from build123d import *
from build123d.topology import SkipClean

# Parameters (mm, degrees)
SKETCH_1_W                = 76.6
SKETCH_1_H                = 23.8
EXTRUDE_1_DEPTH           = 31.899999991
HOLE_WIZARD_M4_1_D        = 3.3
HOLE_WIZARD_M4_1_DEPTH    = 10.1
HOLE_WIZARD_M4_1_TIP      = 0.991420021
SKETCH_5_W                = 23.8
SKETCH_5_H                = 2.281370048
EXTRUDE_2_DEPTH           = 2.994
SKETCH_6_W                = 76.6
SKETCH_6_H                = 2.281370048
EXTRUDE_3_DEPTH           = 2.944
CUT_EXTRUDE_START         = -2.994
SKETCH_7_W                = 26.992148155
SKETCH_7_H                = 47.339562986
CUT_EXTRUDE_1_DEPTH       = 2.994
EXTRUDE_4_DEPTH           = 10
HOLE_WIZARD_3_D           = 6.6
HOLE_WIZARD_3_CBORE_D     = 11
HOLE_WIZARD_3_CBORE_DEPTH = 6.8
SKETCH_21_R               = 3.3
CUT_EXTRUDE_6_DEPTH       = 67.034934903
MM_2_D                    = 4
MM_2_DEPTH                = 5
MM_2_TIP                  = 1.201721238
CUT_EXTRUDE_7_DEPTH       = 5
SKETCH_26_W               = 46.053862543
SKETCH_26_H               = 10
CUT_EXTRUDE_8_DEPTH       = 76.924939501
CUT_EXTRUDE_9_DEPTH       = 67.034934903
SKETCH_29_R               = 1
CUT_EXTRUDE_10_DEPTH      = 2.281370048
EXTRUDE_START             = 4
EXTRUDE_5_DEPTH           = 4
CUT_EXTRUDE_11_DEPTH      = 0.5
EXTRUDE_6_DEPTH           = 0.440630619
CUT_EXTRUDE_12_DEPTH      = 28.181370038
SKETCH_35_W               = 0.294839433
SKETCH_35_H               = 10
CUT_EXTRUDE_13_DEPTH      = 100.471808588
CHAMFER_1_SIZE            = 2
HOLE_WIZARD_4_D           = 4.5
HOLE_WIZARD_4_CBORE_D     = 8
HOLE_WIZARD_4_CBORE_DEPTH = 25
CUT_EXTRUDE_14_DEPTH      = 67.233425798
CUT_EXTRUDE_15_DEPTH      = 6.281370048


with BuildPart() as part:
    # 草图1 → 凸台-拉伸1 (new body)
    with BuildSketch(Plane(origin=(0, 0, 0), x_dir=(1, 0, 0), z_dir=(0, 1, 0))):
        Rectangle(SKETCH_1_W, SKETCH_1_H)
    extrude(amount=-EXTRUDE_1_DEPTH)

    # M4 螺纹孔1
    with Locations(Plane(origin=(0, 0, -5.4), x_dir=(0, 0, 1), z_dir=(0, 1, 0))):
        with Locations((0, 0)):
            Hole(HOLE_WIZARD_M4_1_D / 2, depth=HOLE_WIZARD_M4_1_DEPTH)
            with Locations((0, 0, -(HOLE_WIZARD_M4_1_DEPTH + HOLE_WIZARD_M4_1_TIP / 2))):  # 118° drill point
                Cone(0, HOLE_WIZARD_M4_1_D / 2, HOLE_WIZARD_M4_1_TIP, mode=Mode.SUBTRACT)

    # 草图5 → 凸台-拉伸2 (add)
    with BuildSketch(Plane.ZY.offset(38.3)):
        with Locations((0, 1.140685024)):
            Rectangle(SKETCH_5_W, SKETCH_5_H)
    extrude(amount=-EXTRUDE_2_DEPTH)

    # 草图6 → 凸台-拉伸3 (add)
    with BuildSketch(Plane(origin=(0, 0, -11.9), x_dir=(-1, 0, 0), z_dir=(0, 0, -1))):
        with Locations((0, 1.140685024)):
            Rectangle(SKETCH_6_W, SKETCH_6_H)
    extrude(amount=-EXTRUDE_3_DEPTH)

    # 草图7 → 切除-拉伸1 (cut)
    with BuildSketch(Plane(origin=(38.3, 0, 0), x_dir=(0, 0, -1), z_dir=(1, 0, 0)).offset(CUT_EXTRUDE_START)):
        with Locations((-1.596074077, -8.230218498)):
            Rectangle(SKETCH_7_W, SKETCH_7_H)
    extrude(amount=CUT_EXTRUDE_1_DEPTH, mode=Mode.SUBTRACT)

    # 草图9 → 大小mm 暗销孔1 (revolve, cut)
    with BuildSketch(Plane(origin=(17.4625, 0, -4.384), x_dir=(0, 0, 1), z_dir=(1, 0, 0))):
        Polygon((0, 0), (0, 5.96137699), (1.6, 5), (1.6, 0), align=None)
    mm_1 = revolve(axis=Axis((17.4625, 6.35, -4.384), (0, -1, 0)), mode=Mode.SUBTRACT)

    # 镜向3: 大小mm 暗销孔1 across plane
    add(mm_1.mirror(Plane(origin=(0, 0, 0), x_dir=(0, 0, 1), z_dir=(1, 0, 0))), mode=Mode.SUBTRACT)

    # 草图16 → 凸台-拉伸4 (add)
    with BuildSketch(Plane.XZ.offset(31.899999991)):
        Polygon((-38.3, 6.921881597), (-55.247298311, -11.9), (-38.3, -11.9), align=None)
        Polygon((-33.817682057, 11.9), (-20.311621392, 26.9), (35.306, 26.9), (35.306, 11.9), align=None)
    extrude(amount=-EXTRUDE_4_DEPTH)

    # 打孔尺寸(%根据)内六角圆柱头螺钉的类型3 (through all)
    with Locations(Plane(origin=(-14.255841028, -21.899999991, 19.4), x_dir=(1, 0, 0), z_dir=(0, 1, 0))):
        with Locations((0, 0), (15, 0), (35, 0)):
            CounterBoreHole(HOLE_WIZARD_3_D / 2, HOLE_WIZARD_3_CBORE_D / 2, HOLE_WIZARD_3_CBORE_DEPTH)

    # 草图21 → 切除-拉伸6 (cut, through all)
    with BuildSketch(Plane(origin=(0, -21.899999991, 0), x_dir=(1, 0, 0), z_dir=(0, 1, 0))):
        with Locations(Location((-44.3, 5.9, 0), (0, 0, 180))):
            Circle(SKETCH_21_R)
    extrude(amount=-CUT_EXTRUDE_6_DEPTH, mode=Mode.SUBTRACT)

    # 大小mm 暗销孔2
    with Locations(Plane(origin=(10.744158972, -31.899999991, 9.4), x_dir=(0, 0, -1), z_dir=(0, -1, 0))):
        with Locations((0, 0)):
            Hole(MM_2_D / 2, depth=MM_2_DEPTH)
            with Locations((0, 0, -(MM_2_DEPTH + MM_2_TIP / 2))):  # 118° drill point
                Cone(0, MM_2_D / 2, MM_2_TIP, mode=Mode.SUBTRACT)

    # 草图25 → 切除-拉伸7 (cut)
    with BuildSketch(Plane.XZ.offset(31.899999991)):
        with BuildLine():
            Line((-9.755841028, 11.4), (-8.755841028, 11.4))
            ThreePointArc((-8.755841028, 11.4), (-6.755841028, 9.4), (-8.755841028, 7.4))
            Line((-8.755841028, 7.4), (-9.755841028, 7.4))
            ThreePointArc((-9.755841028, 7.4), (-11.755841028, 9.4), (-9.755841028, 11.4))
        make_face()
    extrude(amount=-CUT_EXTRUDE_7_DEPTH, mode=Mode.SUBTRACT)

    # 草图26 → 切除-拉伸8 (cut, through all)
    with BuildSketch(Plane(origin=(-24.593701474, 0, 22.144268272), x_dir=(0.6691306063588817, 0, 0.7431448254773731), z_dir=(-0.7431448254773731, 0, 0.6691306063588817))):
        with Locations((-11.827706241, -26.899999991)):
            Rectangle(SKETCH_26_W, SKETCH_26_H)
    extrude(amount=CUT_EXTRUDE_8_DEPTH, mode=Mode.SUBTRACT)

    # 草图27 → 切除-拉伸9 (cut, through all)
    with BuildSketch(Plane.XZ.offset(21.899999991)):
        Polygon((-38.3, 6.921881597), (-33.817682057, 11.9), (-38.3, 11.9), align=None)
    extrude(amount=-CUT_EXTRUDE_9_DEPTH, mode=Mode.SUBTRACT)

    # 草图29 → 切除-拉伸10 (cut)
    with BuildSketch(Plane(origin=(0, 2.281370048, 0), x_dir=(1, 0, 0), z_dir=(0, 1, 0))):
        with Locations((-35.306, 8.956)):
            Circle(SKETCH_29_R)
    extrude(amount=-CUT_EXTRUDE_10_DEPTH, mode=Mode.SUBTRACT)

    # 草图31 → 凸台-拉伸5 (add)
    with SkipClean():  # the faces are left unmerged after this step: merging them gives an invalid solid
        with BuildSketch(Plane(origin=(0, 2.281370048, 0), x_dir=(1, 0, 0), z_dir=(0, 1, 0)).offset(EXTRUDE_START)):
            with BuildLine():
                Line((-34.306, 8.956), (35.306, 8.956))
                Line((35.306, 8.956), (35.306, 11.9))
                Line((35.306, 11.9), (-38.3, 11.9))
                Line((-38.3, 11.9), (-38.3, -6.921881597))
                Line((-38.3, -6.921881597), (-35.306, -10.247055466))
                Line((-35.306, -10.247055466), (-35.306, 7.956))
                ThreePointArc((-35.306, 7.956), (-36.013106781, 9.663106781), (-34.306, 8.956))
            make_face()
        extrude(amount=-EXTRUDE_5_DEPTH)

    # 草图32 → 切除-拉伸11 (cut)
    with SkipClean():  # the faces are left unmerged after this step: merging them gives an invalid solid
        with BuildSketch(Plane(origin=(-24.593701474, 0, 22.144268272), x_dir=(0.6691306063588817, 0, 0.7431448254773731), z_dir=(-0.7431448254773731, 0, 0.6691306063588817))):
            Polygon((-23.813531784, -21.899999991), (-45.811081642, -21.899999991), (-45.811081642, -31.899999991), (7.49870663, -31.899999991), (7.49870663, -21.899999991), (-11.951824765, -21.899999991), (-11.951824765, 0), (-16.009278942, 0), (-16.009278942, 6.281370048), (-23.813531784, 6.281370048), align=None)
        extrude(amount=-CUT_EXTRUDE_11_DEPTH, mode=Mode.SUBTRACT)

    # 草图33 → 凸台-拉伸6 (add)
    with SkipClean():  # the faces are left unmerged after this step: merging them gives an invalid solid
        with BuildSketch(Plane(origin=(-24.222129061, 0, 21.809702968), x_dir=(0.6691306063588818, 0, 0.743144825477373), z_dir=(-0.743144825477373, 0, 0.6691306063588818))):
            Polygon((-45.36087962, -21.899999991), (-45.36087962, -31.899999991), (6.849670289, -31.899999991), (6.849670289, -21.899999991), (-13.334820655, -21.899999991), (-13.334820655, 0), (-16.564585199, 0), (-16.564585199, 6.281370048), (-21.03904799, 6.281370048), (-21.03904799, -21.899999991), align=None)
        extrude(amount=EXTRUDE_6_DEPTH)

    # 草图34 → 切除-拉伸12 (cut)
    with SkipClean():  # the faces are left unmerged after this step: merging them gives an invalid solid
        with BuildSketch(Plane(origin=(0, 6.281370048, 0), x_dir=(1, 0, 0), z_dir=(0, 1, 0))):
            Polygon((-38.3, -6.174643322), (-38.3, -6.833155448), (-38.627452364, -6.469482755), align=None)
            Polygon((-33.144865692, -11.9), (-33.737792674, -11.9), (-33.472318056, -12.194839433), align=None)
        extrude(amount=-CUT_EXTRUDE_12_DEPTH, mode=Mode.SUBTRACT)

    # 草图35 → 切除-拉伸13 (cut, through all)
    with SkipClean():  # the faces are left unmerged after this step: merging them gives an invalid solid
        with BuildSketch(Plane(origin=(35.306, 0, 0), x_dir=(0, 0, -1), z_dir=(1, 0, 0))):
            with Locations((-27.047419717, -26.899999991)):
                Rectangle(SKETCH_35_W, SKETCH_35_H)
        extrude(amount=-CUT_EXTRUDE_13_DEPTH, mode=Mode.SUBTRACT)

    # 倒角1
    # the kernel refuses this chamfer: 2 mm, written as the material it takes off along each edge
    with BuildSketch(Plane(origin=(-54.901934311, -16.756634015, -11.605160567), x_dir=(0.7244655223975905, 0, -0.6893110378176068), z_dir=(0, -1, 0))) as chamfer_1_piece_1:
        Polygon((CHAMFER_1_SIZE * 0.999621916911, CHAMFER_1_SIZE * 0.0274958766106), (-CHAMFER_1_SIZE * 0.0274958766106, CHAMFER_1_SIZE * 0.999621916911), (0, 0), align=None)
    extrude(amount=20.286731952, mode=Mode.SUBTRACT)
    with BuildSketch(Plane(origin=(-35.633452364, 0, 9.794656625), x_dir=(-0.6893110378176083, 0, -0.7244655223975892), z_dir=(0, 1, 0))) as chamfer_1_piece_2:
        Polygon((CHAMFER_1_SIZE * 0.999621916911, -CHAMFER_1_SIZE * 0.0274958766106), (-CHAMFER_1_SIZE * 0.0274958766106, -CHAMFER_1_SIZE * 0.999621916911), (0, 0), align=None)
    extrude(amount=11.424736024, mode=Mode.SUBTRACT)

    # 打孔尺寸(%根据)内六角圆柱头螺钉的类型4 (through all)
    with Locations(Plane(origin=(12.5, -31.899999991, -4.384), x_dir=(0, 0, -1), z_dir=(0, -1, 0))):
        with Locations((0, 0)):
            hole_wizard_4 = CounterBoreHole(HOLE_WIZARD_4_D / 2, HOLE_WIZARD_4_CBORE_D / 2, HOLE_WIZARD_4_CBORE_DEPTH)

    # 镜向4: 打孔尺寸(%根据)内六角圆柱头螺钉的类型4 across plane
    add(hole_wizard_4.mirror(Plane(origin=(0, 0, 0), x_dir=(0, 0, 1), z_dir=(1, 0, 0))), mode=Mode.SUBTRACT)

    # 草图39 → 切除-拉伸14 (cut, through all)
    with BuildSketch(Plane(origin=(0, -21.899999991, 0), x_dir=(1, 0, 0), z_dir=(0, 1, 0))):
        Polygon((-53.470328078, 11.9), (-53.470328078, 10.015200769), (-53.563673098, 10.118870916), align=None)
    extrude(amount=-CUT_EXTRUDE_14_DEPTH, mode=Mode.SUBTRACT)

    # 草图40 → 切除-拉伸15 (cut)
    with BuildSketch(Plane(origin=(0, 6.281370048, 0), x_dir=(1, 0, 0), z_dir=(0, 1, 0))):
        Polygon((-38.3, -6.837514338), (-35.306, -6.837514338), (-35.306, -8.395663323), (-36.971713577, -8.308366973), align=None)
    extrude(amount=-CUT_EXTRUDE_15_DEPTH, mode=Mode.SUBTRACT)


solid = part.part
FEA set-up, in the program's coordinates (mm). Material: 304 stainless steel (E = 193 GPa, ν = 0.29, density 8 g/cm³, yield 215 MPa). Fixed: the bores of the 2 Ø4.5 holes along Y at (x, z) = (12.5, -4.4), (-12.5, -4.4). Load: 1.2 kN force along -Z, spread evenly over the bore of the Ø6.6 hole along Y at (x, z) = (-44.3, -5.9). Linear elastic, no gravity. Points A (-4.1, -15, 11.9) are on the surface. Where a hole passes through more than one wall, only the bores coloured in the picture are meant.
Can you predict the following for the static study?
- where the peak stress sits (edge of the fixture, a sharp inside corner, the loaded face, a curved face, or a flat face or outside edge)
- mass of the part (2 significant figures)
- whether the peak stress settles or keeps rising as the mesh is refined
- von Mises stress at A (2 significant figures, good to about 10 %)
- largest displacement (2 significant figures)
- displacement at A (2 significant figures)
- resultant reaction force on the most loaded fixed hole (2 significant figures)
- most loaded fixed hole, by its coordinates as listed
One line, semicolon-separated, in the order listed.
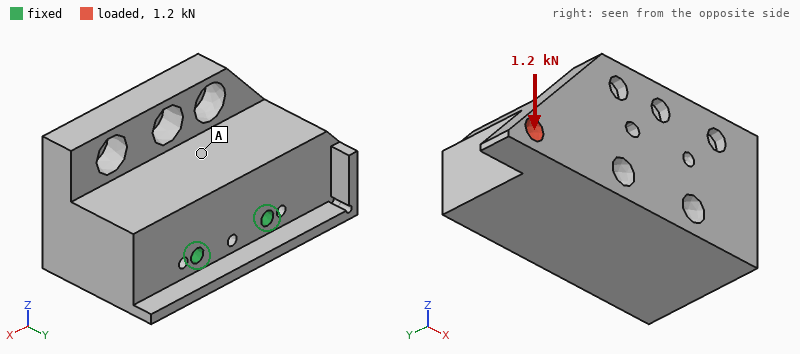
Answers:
edge of the fixture; 500 g; keeps rising; 12 MPa; 28 µm; 8.3 µm; 2.5 kN; (-12.5, -4.4)
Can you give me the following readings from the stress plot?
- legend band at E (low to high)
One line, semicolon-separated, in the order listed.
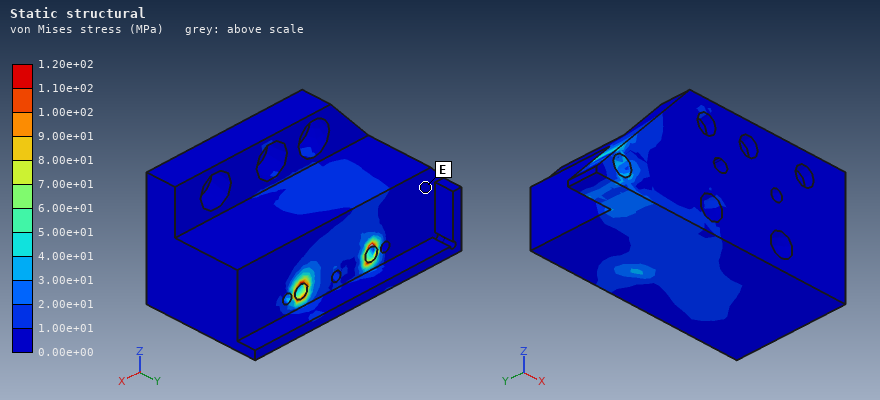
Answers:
0.00e+00 to 1.00e+01 MPa
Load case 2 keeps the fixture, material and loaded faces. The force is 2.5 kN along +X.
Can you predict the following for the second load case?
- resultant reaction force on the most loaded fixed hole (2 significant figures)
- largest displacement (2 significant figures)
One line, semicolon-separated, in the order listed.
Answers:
2.4 kN; 15 µm
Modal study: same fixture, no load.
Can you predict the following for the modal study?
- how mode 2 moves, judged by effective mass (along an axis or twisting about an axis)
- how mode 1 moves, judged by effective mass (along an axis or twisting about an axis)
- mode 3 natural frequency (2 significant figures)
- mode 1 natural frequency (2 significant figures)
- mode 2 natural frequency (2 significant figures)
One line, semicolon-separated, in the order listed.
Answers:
along X; along Z; 6000 Hz; 3000 Hz; 5700 Hz
